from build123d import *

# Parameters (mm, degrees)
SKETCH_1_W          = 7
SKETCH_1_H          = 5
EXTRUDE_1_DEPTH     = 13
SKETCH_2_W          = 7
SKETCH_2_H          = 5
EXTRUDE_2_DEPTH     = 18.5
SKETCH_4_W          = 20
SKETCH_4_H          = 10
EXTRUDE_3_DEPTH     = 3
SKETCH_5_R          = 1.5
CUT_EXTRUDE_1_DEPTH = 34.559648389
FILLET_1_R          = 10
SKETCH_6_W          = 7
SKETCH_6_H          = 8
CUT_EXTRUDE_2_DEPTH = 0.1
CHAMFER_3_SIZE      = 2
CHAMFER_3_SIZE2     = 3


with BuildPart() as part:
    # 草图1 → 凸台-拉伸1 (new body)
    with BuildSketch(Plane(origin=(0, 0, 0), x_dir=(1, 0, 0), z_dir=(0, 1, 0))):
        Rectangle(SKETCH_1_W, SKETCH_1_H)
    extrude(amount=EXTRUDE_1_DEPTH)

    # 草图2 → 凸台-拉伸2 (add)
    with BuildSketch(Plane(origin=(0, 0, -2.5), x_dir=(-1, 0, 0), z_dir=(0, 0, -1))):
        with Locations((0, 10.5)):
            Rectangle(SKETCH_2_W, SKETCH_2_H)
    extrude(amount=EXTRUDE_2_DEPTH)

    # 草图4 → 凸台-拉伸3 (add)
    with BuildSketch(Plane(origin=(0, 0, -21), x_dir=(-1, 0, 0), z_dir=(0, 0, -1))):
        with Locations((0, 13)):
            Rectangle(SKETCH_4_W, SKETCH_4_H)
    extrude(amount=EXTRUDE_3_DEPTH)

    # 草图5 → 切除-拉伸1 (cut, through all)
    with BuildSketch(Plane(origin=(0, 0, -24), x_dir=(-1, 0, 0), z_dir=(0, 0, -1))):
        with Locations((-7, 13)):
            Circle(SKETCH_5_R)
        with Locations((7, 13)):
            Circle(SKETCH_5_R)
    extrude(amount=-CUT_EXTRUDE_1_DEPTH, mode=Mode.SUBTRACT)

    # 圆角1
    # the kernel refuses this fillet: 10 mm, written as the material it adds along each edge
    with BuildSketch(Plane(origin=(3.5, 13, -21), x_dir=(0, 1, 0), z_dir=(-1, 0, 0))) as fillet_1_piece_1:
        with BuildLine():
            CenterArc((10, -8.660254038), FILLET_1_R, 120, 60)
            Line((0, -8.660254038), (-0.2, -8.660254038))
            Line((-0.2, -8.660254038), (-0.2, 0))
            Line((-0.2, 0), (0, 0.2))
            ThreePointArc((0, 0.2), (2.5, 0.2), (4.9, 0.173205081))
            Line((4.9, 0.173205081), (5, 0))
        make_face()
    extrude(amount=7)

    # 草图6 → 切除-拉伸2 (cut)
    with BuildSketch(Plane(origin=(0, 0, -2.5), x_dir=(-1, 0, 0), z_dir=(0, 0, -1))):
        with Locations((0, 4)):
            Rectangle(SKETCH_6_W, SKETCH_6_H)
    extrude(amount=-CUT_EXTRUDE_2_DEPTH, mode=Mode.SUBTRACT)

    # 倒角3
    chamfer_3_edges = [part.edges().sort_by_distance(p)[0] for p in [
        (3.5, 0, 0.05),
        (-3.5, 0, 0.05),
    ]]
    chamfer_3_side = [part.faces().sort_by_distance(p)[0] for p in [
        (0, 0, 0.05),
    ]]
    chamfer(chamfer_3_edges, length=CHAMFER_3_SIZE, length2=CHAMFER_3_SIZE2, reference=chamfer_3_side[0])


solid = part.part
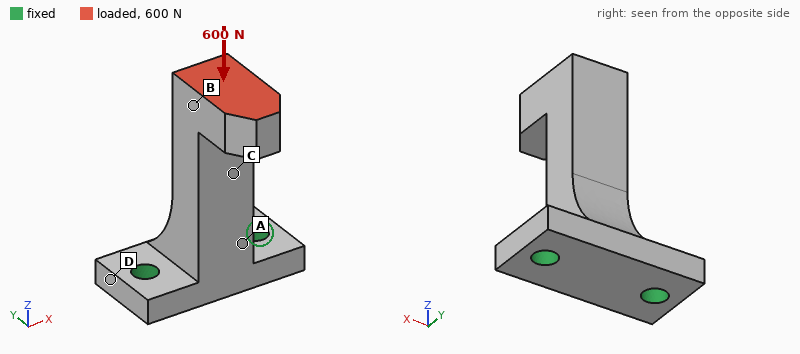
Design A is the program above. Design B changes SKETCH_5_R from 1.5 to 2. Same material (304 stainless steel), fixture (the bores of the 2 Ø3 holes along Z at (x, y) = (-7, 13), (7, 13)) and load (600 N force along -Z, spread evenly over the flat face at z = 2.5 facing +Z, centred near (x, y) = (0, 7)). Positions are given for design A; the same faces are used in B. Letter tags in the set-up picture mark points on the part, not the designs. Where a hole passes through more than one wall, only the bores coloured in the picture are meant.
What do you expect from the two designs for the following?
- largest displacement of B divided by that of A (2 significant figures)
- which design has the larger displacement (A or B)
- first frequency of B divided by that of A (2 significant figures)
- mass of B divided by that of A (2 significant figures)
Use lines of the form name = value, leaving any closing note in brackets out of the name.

largest displacement of B divided by that of A = 0.91
which design has the larger displacement = A
first frequency of B divided by that of A = 1.1
mass of B divided by that of A = 0.98
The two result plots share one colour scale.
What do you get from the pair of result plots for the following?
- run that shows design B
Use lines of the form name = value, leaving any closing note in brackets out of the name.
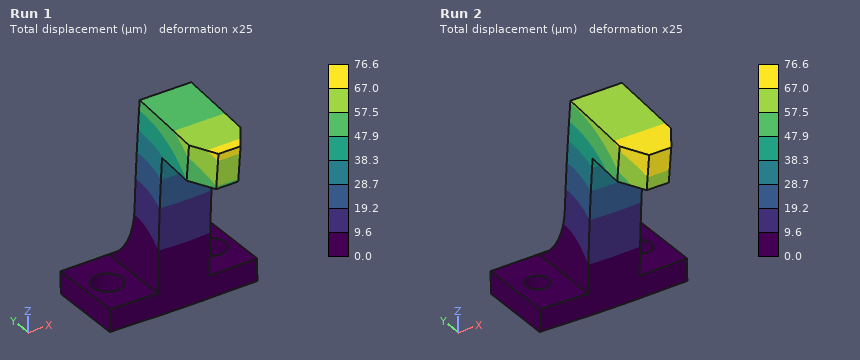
run that shows design B = Run 1
